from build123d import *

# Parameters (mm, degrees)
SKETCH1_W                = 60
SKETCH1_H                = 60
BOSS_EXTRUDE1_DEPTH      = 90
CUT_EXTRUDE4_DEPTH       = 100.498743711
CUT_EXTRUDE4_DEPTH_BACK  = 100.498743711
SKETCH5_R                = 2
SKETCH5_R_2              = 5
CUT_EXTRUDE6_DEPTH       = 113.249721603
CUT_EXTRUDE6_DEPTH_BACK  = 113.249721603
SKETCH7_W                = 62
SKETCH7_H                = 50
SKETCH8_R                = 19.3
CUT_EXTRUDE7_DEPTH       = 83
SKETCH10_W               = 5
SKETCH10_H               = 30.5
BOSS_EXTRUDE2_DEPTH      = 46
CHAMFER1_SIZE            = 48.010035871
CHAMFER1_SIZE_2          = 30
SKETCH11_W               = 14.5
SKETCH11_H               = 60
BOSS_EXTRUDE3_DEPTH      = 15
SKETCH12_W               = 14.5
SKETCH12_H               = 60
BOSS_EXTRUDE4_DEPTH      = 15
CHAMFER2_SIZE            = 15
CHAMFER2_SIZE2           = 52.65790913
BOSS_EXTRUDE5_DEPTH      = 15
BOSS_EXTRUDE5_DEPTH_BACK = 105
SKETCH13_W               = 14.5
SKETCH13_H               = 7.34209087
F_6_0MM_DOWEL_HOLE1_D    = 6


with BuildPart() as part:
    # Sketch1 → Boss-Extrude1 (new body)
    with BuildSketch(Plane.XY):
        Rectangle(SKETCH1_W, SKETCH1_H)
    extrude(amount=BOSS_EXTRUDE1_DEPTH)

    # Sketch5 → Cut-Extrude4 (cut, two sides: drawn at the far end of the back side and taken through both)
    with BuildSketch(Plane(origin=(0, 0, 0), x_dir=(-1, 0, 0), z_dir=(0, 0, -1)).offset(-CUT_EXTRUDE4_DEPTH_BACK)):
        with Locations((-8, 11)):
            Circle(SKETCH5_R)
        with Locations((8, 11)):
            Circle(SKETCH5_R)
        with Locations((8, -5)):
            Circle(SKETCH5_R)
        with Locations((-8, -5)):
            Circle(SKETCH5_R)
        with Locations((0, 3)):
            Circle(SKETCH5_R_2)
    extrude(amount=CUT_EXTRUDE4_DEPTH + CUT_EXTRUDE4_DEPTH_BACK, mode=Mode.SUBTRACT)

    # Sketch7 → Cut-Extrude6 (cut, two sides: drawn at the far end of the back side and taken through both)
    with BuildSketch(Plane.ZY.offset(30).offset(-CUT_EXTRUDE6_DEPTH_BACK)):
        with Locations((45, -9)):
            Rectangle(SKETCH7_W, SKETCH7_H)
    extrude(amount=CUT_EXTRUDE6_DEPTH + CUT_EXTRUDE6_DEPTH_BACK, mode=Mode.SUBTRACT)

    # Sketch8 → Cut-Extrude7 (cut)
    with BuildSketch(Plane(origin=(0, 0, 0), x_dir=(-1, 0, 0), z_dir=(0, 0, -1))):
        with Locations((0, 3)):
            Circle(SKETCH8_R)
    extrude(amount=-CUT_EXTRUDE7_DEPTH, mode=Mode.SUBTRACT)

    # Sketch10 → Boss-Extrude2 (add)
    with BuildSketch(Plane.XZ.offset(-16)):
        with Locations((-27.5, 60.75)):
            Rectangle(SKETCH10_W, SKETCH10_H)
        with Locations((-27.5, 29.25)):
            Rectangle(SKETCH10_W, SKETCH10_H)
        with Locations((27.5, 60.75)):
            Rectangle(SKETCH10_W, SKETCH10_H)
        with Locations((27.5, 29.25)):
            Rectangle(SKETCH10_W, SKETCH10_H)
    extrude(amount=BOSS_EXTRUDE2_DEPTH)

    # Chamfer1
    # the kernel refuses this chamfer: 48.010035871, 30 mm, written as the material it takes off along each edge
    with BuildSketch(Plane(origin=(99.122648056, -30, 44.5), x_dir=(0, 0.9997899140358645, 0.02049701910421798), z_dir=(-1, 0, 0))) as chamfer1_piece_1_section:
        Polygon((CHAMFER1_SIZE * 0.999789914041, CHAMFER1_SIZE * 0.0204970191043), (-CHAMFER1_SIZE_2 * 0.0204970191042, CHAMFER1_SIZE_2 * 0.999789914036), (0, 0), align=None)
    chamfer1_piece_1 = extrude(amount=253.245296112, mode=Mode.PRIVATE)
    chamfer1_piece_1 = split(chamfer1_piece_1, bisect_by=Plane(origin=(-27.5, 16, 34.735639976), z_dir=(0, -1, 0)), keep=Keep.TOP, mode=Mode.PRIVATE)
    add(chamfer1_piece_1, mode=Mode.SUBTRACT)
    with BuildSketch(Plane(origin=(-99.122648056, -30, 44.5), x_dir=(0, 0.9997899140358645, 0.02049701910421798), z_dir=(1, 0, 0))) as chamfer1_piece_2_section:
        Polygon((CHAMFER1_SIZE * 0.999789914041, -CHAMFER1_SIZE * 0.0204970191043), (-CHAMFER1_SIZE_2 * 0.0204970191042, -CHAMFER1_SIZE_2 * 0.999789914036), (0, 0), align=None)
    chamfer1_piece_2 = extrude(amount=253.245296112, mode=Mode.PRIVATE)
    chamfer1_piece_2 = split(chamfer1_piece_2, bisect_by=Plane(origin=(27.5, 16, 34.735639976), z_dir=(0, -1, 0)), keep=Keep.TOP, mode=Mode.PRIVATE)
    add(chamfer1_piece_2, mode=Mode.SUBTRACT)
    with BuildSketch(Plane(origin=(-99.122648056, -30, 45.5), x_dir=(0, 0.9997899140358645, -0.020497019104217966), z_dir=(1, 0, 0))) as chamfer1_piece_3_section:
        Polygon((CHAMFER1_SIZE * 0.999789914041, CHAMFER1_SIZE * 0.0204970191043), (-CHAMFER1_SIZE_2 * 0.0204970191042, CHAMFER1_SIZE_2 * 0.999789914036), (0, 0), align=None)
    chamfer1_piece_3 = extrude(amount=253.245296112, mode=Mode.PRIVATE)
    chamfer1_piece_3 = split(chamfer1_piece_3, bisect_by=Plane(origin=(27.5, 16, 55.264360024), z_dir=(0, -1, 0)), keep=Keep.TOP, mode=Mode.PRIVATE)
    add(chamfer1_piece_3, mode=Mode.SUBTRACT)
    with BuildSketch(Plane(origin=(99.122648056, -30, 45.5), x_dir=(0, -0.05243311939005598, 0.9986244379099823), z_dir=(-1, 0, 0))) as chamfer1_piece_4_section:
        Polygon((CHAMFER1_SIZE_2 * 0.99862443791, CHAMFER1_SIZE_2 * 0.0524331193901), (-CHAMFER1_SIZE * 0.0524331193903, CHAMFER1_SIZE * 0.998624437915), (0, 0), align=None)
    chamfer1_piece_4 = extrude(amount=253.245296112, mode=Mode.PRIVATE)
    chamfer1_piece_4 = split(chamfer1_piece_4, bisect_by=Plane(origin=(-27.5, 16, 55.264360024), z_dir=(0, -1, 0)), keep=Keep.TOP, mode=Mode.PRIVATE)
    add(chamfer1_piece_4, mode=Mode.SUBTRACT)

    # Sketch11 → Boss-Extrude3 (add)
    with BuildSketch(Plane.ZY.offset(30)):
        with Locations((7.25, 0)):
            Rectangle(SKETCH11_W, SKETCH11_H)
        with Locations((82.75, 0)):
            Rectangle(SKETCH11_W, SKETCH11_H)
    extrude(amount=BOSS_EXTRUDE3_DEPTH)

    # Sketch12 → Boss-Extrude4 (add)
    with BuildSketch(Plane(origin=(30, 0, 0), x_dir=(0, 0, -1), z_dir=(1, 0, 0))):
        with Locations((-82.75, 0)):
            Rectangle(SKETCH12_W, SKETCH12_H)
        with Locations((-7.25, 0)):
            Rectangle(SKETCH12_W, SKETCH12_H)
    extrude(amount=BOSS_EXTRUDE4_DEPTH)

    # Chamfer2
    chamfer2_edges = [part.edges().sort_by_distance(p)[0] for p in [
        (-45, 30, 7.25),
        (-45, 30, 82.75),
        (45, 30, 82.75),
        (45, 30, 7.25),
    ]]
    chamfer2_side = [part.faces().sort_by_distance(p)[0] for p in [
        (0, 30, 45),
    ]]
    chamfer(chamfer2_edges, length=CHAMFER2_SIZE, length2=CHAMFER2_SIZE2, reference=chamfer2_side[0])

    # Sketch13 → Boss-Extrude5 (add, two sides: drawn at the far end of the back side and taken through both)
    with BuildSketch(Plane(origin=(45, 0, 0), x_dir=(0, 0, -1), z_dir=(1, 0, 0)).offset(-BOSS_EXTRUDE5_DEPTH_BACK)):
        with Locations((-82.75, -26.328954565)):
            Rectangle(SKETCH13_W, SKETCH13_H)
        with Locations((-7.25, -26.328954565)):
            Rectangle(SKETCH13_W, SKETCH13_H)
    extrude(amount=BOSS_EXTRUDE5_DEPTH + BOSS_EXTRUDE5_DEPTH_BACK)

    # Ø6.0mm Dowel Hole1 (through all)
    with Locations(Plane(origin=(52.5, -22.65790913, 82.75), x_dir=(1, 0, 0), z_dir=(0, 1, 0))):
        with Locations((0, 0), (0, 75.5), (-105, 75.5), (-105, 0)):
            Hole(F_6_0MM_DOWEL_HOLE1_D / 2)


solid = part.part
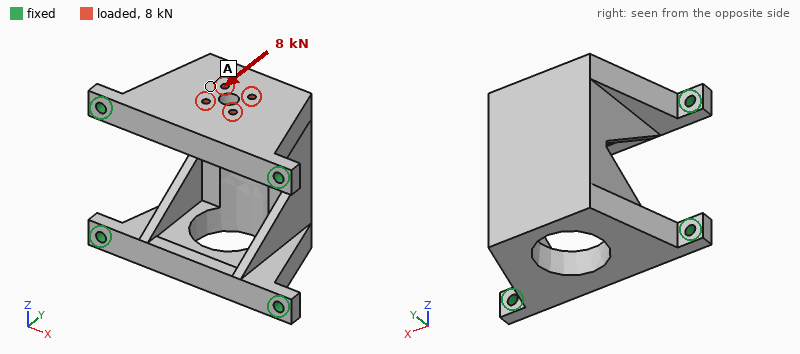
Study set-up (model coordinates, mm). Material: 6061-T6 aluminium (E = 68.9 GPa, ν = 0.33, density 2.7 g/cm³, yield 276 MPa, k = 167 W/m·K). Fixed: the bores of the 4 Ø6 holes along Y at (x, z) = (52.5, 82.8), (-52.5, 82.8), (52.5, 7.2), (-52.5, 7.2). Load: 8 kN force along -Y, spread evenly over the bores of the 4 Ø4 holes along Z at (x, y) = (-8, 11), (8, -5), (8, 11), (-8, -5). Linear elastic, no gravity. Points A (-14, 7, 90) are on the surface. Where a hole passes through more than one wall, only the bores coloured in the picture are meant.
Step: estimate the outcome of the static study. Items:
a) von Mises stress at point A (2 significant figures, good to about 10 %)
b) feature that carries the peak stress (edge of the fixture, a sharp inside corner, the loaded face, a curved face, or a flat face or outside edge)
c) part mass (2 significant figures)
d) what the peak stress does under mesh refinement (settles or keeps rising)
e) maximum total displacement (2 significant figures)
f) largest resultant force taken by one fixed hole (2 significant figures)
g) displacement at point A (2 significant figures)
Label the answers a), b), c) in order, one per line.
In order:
a) 20 MPa
b) edge of the fixture
c) 460 g
d) keeps rising
e) 59 µm
f) 5.1 kN
g) 51 µm
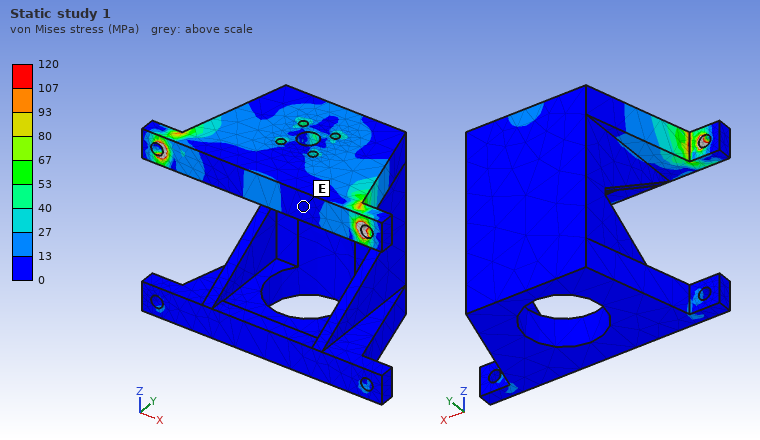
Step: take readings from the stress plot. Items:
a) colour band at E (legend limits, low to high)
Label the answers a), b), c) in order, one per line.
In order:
a) 0 to 13 MPa
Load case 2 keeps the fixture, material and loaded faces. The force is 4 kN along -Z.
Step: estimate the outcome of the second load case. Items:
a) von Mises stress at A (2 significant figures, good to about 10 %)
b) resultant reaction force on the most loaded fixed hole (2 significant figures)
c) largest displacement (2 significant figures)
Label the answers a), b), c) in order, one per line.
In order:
a) 17 MPa
b) 1.5 kN
c) 76 µm
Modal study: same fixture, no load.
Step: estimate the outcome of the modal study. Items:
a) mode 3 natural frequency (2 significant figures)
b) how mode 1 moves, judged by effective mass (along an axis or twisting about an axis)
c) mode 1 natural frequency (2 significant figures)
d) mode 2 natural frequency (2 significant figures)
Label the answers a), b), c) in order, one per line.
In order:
a) 4600 Hz
b) along Z
c) 2300 Hz
d) 4500 Hz
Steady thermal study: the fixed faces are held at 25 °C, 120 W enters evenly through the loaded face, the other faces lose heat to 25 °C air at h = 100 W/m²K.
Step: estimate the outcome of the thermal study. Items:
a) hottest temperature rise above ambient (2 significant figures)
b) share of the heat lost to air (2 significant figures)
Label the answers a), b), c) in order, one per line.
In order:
a) 40 K
b) 51 %
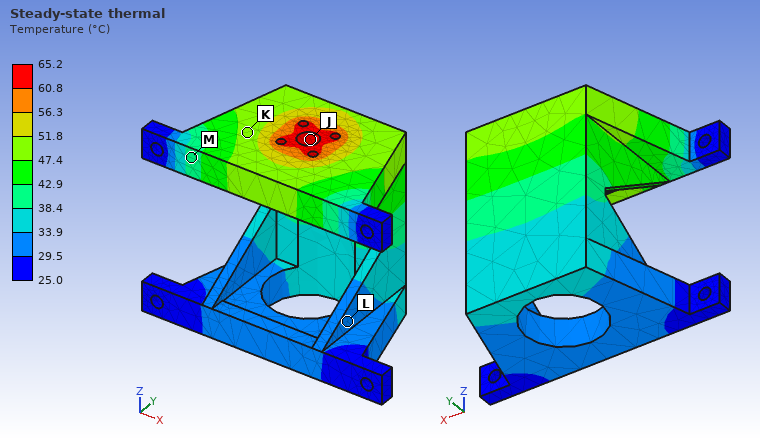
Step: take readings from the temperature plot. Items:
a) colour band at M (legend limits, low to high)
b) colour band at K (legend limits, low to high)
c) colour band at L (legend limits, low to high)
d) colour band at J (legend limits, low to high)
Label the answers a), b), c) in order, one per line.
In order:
a) 38.4 to 42.9 °C
b) 47.4 to 51.8 °C
c) 29.5 to 33.9 °C
d) 60.8 to 65.2 °C
